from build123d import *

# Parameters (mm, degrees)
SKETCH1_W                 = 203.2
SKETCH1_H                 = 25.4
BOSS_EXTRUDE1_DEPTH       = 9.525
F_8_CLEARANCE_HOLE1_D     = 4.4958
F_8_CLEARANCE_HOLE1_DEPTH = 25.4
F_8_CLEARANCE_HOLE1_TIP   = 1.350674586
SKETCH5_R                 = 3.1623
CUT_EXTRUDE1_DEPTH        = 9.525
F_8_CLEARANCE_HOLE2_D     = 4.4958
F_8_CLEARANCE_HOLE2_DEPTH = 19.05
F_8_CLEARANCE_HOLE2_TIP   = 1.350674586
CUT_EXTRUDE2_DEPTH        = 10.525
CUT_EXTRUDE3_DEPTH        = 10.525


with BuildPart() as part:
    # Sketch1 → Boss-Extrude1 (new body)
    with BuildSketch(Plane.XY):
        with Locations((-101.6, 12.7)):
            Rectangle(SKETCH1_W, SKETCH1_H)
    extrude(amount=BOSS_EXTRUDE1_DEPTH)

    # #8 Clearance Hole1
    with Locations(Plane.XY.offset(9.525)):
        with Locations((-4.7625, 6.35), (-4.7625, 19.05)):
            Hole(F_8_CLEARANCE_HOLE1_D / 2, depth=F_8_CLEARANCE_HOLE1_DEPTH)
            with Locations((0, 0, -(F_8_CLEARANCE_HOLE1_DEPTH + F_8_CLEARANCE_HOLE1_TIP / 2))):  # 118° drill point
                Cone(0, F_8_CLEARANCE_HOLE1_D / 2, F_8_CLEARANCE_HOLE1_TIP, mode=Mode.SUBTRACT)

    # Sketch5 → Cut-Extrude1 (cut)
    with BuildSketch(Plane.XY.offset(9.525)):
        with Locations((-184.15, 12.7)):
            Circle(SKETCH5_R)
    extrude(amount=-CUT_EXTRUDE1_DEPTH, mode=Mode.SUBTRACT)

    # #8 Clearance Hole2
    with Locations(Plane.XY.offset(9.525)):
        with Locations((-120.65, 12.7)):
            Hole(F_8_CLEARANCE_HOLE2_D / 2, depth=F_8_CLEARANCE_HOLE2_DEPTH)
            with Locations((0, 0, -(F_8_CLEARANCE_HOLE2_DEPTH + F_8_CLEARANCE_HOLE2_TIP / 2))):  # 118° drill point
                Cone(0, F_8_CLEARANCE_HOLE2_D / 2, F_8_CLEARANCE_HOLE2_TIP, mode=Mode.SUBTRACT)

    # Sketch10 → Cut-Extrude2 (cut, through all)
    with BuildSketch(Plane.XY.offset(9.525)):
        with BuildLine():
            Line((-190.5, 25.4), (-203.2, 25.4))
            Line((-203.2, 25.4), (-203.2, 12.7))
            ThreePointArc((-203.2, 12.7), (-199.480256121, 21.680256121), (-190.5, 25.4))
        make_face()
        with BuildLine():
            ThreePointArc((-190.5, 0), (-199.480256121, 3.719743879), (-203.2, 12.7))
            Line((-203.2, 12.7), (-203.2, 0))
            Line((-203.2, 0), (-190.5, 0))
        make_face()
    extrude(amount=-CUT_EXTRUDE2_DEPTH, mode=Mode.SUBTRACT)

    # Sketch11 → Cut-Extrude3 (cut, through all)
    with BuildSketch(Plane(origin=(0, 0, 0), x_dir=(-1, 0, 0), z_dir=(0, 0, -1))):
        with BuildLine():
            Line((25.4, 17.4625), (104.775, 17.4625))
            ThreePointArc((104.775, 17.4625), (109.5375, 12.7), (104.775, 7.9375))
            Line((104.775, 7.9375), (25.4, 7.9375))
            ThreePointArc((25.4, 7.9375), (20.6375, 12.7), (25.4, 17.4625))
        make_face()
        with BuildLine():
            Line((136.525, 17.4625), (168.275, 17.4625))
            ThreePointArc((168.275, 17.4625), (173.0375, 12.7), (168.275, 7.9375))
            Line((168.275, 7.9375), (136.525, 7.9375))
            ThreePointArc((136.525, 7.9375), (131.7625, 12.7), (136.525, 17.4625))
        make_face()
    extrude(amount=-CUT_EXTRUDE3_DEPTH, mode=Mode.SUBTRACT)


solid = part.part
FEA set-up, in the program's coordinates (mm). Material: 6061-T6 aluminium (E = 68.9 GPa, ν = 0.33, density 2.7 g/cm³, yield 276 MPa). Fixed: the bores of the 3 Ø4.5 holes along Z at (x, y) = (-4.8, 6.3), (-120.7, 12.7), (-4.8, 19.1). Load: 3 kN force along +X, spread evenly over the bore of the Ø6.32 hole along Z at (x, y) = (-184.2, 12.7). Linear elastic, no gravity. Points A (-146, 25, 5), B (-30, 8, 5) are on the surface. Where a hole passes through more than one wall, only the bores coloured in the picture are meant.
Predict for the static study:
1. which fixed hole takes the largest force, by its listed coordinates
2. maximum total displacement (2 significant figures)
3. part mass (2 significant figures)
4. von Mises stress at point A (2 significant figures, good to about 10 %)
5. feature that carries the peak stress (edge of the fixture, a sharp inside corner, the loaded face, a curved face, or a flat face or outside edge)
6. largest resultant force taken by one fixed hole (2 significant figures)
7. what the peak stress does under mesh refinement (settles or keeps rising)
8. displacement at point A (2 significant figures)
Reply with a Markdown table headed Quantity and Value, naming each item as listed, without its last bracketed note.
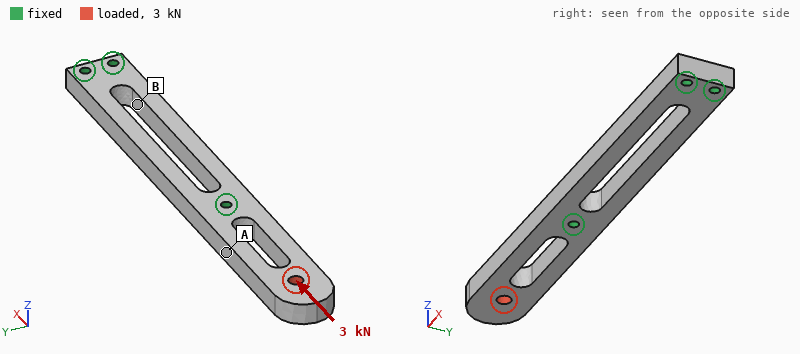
| Quantity | Value |
|---|---|
| which fixed hole takes the largest force, by its listed coordinates | (-120.7, 12.7) |
| maximum total displacement | 21 µm |
| part mass | 98 g |
| von Mises stress at point A | 14 MPa |
| feature that carries the peak stress | edge of the fixture |
| largest resultant force taken by one fixed hole | 2.8 kN |
| what the peak stress does under mesh refinement | keeps rising |
| displacement at point A | 11 µm |
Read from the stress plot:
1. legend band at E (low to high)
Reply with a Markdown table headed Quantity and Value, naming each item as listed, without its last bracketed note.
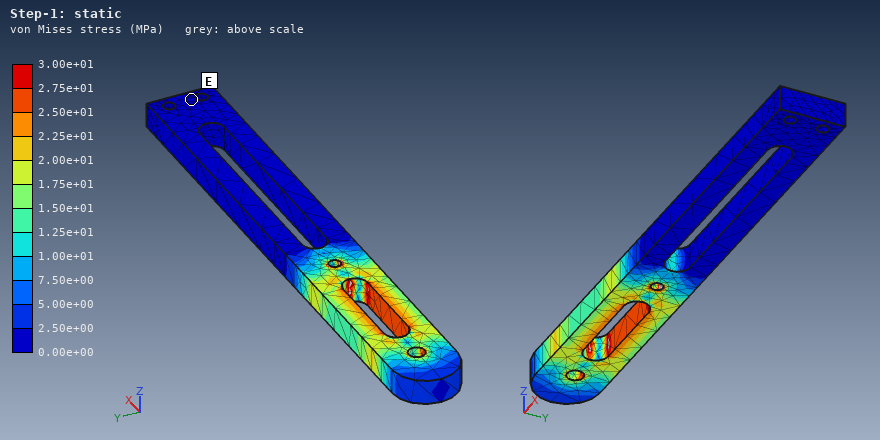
| Quantity | Value |
|---|---|
| legend band at E | 0.00e+00 to 2.50e+00 MPa |
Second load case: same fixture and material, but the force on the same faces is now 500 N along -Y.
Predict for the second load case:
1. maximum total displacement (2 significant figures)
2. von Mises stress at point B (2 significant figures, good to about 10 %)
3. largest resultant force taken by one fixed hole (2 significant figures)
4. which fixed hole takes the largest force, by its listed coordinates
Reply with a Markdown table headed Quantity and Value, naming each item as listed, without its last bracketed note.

| Quantity | Value |
|---|---|
| maximum total displacement | 0.24 mm |
| von Mises stress at point B | 13 MPa |
| largest resultant force taken by one fixed hole | 550 N |
| which fixed hole takes the largest force, by its listed coordinates | (-120.7, 12.7) |
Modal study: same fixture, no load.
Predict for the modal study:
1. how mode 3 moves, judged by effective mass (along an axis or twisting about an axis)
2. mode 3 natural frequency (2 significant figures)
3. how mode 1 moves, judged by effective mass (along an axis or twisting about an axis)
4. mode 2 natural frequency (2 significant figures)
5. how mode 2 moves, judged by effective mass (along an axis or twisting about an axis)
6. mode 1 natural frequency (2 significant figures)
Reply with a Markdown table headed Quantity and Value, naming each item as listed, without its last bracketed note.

| Quantity | Value |
|---|---|
| how mode 3 moves, judged by effective mass | along Z |
| mode 3 natural frequency | 3900 Hz |
| how mode 1 moves, judged by effective mass | along Z |
| mode 2 natural frequency | 1700 Hz |
| how mode 2 moves, judged by effective mass | along Y |
| mode 1 natural frequency | 1000 Hz |
